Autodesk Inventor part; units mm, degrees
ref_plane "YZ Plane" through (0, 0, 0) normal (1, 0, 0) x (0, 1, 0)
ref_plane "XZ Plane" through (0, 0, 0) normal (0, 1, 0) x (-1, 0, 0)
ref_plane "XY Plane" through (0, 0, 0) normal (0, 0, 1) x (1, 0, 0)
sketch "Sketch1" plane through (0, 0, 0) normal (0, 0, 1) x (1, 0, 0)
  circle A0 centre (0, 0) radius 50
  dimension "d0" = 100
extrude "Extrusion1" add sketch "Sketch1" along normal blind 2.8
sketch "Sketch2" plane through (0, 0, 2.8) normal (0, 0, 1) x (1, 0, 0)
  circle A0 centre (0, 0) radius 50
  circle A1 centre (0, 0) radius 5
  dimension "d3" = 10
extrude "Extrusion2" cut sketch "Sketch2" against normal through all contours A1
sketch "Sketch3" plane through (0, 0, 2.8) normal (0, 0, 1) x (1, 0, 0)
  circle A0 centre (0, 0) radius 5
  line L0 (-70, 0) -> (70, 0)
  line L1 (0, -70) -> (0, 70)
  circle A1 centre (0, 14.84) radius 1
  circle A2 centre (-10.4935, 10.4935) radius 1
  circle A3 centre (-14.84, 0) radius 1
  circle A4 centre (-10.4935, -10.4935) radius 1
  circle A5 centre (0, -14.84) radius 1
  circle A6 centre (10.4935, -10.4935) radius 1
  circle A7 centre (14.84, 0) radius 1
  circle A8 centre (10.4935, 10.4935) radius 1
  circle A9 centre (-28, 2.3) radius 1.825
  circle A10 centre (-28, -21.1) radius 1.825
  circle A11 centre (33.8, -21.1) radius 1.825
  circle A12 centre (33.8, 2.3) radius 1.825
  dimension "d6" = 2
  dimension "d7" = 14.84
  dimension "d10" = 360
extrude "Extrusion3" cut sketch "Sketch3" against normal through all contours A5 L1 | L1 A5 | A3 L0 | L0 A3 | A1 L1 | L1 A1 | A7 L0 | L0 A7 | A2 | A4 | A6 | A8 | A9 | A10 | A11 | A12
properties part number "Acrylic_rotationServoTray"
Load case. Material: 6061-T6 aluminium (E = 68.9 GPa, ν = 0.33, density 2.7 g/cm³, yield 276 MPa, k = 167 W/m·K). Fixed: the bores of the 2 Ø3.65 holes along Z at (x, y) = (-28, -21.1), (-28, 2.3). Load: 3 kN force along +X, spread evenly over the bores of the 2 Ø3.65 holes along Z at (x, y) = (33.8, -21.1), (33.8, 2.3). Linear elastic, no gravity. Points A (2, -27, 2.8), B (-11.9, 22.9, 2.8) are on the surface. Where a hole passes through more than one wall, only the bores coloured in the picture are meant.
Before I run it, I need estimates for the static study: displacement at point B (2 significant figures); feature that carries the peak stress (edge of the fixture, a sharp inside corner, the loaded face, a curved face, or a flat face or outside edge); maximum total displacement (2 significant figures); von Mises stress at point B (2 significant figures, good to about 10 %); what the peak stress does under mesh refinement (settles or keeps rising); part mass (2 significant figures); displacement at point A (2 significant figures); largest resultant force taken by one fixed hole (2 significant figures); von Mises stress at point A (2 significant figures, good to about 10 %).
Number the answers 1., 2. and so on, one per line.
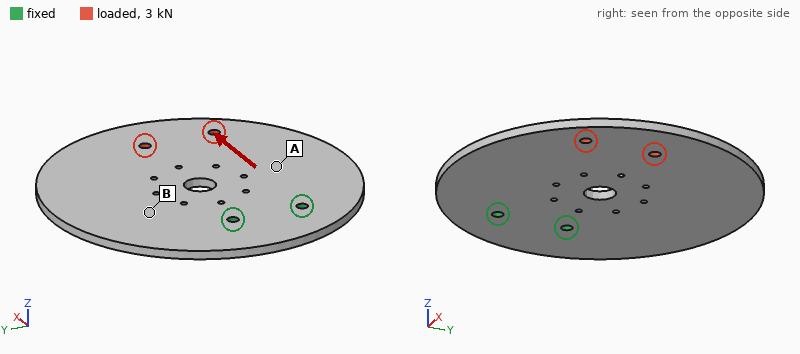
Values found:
1. 11 µm
2. edge of the fixture
3. 25 µm
4. 7.4 MPa
5. keeps rising
6. 58 g
7. 12 µm
8. 1.5 kN
9. 18 MPa
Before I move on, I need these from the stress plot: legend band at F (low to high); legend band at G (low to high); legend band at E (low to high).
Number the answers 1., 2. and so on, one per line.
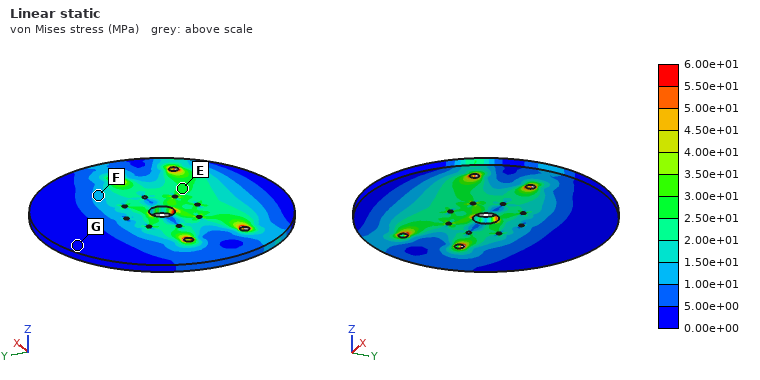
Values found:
1. 1.00e+01 to 1.50e+01 MPa
2. 0.00e+00 to 5.00e+00 MPa
3. 2.50e+01 to 3.00e+01 MPa
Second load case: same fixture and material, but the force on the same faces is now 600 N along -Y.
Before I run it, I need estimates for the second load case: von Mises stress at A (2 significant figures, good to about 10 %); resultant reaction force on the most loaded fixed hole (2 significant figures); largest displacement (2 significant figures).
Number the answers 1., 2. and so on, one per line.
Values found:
1. 7.6 MPa
2. 1.5 kN
3. 56 µm
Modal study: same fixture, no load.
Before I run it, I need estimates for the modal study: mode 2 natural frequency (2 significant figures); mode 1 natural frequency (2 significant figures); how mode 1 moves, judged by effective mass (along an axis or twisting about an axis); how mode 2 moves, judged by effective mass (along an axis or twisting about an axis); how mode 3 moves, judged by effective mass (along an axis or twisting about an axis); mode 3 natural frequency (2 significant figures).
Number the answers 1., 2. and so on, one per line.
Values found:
1. 740 Hz
2. 390 Hz
3. along Z
4. twisting about X
5. along Z
6. 1500 Hz
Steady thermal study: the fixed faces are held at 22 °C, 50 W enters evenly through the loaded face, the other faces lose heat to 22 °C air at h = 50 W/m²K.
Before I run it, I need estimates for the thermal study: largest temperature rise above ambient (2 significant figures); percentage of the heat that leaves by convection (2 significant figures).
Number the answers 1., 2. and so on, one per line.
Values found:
1. 80 K
2. 49 %
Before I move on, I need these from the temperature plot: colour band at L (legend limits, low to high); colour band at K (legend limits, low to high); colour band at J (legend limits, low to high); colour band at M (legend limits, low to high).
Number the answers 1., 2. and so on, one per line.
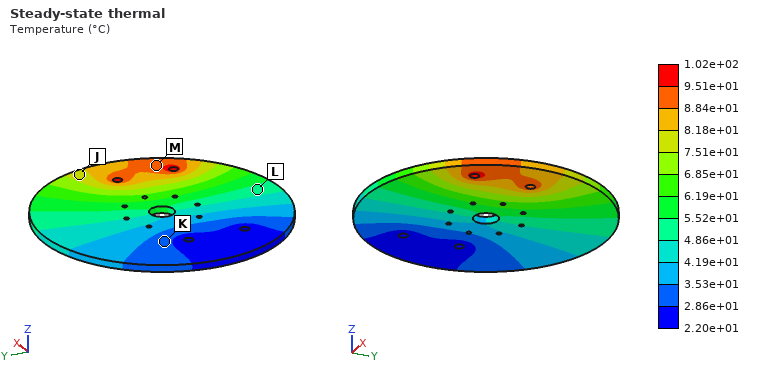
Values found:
1. 4.86e+01 to 5.52e+01 °C
2. 2.86e+01 to 3.53e+01 °C
3. 7.51e+01 to 8.18e+01 °C
4. 8.84e+01 to 9.51e+01 °C
